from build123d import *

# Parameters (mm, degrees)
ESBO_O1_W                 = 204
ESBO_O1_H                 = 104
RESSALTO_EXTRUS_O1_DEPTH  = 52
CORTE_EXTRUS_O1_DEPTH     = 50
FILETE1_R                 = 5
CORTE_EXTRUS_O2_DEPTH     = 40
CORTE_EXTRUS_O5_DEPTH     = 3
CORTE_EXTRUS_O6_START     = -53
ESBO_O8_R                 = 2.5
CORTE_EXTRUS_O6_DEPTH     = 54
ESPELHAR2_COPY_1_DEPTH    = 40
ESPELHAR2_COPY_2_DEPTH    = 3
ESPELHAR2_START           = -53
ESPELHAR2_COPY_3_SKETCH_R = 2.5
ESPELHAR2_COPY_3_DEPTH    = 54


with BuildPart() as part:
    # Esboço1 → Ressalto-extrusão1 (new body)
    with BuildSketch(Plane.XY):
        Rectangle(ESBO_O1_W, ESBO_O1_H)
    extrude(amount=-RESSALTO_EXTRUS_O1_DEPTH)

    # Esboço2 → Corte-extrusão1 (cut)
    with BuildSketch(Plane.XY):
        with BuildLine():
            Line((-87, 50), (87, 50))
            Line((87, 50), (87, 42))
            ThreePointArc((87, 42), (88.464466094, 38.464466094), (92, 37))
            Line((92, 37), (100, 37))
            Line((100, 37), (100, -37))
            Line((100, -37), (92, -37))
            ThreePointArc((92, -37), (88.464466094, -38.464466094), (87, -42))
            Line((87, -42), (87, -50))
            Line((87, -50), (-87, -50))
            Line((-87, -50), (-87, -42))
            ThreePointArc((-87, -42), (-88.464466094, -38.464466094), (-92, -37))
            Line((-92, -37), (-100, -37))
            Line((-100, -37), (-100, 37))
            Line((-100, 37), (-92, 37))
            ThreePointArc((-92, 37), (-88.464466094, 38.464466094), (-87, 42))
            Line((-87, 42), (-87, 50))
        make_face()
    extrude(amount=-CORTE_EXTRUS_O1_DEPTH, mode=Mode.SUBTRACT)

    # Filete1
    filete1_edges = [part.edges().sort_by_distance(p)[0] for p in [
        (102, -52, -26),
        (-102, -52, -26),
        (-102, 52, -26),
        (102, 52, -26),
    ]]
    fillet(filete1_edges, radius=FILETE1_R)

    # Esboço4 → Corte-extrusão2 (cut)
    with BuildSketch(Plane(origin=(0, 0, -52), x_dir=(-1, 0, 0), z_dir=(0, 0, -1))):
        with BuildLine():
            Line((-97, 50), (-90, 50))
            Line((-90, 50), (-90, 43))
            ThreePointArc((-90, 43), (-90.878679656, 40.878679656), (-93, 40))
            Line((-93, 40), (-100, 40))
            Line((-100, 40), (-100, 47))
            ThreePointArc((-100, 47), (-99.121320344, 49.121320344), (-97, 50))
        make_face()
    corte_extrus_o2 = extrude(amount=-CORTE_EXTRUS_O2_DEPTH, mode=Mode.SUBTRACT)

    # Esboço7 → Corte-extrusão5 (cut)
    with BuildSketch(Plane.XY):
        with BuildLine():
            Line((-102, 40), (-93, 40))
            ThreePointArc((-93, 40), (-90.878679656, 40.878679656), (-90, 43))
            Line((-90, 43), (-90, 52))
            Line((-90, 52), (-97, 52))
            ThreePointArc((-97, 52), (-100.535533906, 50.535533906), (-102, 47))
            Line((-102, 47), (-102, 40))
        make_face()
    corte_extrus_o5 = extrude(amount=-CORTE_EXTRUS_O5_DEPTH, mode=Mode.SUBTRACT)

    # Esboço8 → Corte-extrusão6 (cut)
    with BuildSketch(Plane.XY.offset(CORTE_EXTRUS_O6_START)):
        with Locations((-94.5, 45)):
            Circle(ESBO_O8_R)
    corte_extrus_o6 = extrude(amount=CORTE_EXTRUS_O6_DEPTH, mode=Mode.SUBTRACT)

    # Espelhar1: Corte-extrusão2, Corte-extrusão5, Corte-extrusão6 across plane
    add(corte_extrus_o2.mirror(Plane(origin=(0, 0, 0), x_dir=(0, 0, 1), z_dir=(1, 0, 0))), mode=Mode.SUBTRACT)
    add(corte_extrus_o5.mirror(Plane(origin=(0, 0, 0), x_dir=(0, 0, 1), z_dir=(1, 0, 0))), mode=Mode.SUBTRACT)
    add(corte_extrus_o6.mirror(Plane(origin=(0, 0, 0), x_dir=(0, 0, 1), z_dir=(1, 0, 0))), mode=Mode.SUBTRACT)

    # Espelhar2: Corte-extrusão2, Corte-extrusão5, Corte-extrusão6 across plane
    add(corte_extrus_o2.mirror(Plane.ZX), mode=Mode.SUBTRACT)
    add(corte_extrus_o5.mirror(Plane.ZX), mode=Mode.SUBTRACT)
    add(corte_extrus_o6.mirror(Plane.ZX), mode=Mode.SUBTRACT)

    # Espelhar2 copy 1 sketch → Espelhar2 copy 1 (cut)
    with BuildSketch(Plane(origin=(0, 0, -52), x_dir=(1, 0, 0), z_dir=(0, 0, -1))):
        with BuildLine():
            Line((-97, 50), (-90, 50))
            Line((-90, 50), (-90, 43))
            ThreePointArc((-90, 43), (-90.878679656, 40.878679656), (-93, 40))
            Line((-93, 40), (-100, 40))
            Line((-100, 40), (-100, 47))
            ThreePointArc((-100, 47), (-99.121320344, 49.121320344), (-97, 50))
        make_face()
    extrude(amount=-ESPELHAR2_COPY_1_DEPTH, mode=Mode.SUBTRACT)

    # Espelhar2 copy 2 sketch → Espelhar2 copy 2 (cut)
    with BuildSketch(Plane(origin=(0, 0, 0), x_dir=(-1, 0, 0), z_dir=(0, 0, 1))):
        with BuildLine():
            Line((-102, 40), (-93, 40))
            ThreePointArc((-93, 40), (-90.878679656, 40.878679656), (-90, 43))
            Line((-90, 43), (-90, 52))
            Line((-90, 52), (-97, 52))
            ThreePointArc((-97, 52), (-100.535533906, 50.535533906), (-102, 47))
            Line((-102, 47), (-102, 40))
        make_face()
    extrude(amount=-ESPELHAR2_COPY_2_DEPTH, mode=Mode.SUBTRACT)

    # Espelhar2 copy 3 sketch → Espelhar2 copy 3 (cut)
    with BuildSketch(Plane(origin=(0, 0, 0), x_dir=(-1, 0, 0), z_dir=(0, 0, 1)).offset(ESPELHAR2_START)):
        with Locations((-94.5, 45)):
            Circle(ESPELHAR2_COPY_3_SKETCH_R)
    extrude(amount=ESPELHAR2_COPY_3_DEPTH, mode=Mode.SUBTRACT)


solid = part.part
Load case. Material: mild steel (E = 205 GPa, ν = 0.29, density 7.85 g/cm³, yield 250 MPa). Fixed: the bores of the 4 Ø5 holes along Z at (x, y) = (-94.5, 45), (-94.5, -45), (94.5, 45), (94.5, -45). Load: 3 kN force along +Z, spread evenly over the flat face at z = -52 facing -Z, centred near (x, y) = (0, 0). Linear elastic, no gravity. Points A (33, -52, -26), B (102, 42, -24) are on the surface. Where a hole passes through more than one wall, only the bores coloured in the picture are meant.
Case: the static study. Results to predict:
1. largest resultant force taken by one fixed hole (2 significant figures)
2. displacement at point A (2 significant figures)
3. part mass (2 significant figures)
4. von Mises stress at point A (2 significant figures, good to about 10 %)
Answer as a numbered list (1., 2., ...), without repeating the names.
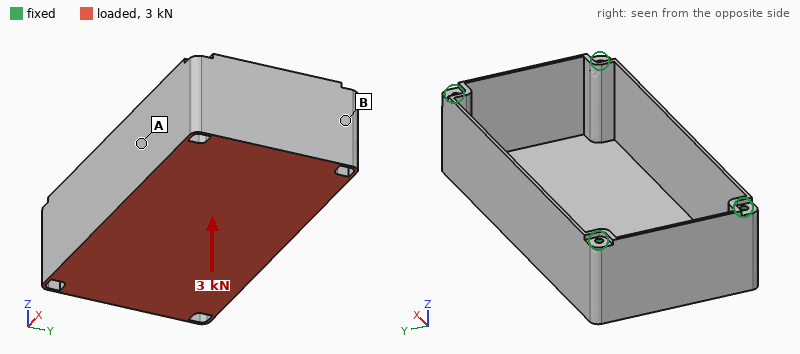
1. 880 N
2. 0.21 mm
3. 920 g
4. 41 MPa
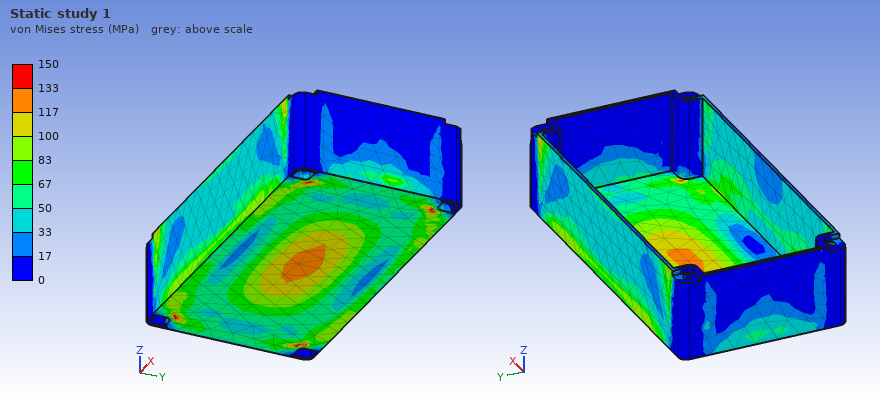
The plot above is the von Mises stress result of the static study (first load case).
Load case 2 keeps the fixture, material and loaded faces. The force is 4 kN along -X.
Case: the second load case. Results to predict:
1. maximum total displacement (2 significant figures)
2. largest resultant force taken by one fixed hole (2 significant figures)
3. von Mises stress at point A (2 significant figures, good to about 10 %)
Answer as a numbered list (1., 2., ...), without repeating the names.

1. 8.2 µm
2. 1.1 kN
3. 9.1 MPa
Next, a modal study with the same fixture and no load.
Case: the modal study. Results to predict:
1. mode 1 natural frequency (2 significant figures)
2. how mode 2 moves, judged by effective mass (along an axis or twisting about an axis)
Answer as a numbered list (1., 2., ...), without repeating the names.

1. 570 Hz
2. along Y
